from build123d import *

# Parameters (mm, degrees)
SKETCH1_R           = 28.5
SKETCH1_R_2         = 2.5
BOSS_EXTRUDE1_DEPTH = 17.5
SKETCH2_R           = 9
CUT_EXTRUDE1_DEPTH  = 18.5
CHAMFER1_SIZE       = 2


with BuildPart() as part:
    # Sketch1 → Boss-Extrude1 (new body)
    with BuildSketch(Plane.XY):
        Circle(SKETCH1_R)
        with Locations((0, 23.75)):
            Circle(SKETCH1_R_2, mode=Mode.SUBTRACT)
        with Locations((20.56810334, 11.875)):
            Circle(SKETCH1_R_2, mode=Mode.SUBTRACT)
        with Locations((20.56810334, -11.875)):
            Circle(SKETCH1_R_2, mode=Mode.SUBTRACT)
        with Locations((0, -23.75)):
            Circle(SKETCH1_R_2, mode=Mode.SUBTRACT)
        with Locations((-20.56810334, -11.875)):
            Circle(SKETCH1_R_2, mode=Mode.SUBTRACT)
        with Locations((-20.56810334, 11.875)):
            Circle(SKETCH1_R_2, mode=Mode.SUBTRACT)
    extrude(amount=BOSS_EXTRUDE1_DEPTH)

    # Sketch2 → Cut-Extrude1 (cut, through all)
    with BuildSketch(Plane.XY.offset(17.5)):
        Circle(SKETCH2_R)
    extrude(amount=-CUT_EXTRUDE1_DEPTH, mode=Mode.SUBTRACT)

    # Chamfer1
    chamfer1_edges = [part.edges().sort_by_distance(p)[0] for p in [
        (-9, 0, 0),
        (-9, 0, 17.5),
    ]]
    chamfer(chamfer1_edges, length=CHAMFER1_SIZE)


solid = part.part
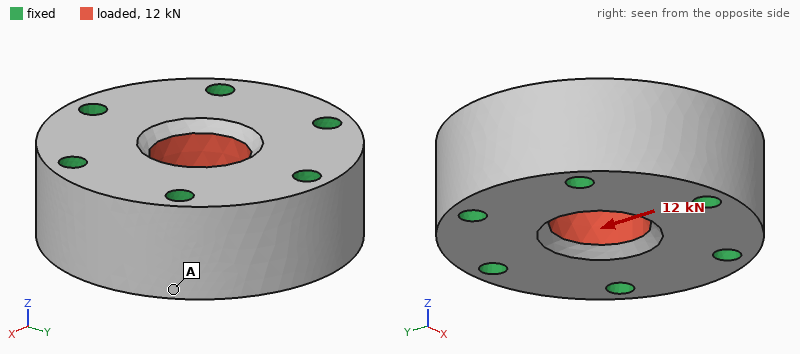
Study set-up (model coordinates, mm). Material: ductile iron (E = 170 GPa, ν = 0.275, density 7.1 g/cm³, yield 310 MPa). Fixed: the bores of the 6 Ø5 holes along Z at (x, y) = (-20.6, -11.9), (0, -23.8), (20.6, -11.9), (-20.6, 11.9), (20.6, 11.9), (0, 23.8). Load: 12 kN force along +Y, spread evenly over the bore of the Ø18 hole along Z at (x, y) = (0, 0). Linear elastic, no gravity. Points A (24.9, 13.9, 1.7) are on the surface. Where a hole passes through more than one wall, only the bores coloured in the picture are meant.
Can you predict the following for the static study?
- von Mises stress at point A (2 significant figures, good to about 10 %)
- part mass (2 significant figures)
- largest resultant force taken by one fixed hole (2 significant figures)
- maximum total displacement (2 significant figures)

2.4 MPa
270 g
3.0 kN
1.3 µm
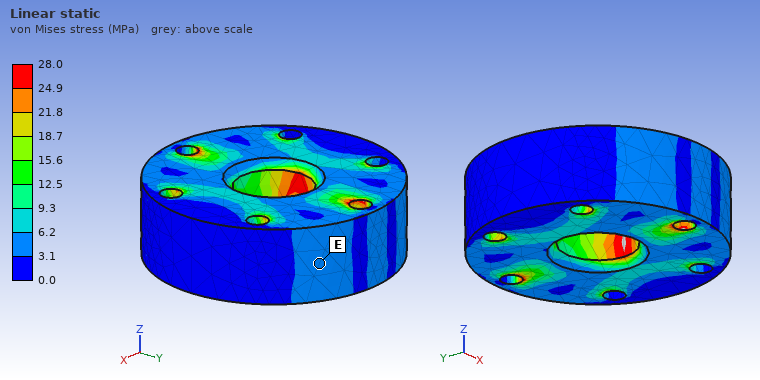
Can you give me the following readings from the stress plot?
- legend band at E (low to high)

3.1 to 6.2 MPa
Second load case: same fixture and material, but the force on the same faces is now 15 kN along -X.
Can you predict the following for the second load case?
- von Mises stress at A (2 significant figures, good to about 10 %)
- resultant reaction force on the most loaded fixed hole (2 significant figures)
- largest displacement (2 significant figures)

5.8 MPa
3.3 kN
1.7 µm
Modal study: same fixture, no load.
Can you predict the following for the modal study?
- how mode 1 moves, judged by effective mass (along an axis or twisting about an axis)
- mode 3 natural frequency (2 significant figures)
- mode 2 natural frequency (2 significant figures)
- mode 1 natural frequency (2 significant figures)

along Z
52 kHz
52 kHz
42 kHz
